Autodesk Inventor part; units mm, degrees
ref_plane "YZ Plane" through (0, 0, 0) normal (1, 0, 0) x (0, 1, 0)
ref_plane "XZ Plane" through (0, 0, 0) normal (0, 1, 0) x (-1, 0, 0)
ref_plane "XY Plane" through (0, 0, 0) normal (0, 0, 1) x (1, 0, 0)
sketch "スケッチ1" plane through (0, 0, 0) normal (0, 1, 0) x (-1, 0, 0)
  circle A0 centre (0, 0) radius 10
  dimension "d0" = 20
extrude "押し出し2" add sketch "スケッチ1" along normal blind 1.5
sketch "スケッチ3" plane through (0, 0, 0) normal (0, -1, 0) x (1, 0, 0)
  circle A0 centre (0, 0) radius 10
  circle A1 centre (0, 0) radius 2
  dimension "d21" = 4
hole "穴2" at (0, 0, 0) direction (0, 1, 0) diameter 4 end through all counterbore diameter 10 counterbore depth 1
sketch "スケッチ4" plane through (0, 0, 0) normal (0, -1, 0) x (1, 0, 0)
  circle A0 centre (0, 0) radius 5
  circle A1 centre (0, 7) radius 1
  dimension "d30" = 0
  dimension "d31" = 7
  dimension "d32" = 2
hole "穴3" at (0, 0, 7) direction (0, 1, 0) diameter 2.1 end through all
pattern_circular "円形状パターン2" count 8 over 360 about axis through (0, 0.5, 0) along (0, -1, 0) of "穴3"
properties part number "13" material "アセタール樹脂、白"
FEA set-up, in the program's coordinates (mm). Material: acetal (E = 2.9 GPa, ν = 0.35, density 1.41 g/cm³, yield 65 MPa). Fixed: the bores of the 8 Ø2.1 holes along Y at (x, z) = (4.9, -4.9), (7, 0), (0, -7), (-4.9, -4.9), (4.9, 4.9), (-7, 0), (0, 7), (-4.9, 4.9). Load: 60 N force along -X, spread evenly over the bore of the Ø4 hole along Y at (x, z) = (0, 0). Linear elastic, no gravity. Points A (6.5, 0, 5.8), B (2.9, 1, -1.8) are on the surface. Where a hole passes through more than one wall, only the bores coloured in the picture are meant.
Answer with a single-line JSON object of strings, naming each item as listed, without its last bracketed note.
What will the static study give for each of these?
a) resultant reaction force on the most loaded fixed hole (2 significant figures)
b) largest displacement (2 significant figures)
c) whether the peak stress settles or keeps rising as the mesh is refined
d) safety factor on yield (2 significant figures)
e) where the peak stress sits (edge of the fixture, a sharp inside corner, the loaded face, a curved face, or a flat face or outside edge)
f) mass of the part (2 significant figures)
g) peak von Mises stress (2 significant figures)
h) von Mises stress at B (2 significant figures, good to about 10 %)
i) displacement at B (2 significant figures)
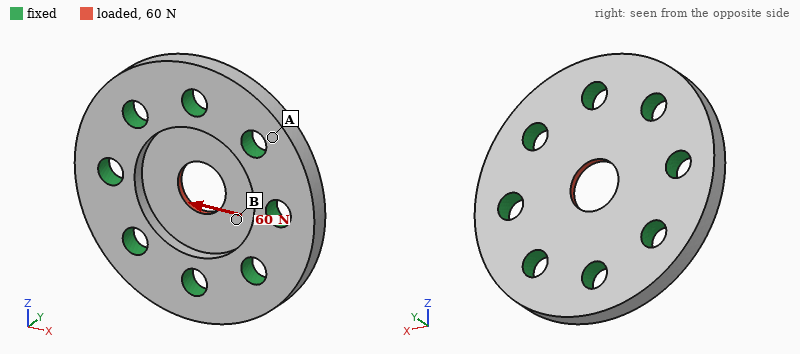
{"resultant reaction force on the most loaded fixed hole": "13 N", "largest displacement": "12 µm", "whether the peak stress settles or keeps rising as the mesh is refined": "settles", "safety factor on yield": "3.9", "where the peak stress sits": "the loaded face", "mass of the part": "0.49 g", "peak von Mises stress": "17 MPa", "von Mises stress at B": "7.7 MPa", "displacement at B": "6.9 µm"}
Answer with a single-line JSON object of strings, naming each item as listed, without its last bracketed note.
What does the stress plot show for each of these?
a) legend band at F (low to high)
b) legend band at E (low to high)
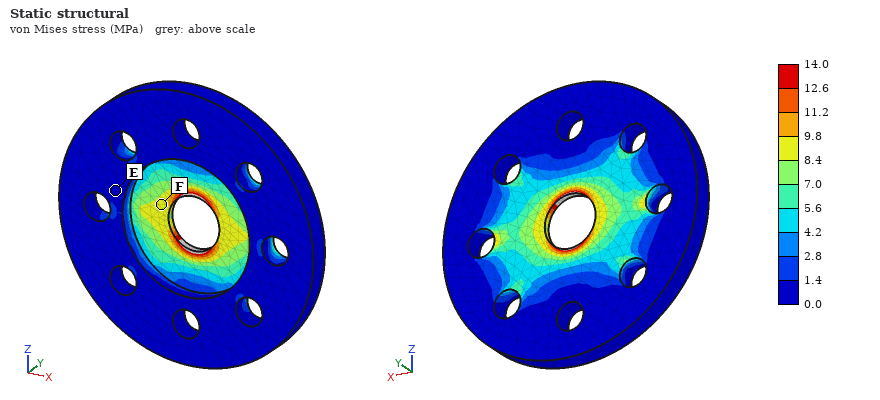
{"legend band at F": "8.4 to 9.8 MPa", "legend band at E": "0.0 to 1.4 MPa"}
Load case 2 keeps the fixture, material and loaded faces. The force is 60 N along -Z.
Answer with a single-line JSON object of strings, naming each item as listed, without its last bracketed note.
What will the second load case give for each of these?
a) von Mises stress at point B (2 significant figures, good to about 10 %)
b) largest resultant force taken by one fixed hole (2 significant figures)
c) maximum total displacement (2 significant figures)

{"von Mises stress at point B": "6.6 MPa", "largest resultant force taken by one fixed hole": "13 N", "maximum total displacement": "12 µm"}
